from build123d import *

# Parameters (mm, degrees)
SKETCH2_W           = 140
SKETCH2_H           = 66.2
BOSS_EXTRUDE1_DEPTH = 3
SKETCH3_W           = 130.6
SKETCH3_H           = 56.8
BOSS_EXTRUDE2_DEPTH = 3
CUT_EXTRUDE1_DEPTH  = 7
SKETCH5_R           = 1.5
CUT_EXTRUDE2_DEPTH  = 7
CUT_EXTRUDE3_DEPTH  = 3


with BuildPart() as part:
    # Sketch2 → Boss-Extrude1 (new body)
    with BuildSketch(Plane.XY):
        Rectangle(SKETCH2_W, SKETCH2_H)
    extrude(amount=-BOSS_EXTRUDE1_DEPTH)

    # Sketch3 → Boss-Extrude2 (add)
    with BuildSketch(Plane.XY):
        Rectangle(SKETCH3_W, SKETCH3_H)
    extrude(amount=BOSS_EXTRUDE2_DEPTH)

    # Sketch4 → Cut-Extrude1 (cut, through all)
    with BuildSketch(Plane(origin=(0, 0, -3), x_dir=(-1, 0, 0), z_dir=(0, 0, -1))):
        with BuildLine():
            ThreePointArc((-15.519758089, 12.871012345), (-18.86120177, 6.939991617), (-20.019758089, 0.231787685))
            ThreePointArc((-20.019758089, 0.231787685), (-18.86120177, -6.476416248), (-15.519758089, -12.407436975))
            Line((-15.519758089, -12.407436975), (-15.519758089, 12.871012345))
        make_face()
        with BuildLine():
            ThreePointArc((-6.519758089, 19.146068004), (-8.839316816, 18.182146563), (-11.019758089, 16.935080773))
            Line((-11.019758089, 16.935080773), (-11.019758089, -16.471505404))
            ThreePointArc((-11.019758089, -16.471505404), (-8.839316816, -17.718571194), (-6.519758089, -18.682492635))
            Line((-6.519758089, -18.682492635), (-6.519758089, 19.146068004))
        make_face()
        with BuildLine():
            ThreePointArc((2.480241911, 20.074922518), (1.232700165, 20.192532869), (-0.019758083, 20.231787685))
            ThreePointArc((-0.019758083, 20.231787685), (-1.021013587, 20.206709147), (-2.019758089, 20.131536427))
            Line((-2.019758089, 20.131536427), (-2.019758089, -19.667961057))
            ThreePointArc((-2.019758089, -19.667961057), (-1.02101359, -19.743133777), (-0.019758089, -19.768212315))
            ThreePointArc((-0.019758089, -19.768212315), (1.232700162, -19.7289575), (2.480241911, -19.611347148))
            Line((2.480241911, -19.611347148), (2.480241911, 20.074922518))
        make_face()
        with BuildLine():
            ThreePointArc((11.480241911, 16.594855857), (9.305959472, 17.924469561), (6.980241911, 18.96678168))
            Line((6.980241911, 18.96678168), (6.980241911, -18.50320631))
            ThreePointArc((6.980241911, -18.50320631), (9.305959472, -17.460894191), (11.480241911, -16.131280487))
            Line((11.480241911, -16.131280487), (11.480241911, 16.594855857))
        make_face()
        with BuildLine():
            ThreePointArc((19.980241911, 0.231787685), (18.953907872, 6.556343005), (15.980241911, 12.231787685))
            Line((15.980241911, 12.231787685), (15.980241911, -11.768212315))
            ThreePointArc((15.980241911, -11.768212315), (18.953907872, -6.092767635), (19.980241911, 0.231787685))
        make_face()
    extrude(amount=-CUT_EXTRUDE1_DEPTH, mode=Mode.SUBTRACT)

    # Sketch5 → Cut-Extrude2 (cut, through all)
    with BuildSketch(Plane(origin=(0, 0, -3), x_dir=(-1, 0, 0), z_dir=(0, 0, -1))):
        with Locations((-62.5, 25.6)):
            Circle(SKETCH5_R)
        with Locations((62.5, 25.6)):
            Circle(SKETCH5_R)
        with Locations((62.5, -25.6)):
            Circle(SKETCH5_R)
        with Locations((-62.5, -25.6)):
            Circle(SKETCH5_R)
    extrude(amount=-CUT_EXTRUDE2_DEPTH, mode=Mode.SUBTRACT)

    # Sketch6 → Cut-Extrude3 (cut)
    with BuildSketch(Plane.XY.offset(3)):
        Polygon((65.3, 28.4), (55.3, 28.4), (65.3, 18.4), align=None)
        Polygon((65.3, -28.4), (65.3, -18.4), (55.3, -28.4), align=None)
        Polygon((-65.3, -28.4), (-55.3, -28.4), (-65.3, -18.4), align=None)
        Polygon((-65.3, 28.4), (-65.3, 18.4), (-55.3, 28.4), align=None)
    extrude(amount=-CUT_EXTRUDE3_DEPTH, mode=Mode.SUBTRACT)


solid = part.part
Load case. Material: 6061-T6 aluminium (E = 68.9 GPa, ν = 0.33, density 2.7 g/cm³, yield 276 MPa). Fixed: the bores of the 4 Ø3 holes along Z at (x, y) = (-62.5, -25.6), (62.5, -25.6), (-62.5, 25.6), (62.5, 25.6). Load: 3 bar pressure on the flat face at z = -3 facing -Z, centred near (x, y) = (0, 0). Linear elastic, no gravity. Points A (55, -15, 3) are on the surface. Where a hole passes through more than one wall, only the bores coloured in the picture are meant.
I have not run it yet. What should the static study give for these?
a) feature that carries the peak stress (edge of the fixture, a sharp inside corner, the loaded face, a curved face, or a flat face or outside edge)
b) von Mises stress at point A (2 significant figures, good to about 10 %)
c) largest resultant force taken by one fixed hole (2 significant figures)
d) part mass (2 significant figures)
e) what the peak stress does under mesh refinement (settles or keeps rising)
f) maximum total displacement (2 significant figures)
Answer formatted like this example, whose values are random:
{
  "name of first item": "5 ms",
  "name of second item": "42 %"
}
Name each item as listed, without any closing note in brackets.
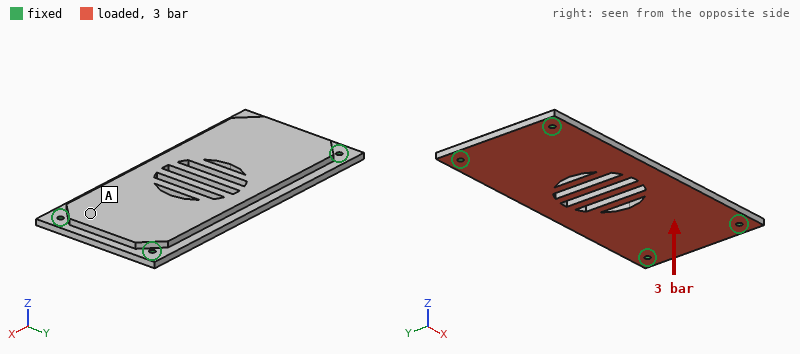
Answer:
{
  "feature that carries the peak stress": "edge of the fixture",
  "von Mises stress at point A": "33 MPa",
  "largest resultant force taken by one fixed hole": "1.4 kN",
  "part mass": "120 g",
  "what the peak stress does under mesh refinement": "keeps rising",
  "maximum total displacement": "0.55 mm"
}
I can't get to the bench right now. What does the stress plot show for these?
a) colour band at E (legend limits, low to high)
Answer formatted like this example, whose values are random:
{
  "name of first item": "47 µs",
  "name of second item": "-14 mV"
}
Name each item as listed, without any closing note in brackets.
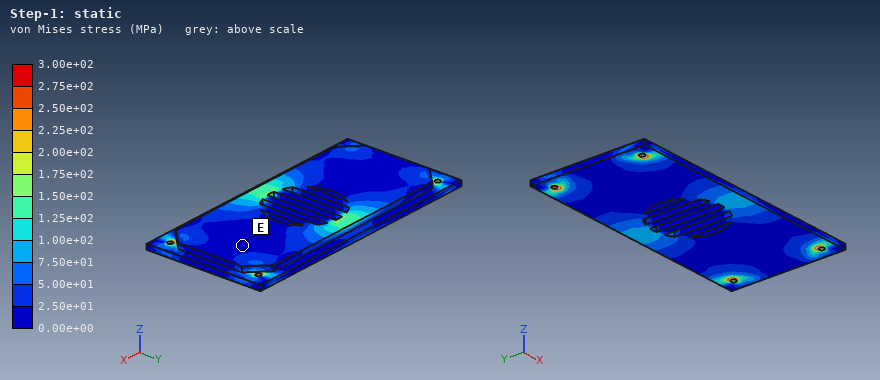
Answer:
{
  "colour band at E": "0.00e+00 to 2.50e+01 MPa"
}
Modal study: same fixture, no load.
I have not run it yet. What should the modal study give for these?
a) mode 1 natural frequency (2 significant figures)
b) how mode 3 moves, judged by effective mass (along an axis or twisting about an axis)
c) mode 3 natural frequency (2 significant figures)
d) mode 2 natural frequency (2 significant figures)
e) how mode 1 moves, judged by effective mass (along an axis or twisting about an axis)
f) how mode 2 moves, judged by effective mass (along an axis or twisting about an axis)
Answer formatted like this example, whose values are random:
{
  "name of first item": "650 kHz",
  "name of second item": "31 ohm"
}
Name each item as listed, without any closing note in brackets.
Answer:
{
  "mode 1 natural frequency": "1100 Hz",
  "how mode 3 moves, judged by effective mass": "twisting about Y",
  "mode 3 natural frequency": "3400 Hz",
  "mode 2 natural frequency": "2700 Hz",
  "how mode 1 moves, judged by effective mass": "along Z",
  "how mode 2 moves, judged by effective mass": "twisting about X"
}
